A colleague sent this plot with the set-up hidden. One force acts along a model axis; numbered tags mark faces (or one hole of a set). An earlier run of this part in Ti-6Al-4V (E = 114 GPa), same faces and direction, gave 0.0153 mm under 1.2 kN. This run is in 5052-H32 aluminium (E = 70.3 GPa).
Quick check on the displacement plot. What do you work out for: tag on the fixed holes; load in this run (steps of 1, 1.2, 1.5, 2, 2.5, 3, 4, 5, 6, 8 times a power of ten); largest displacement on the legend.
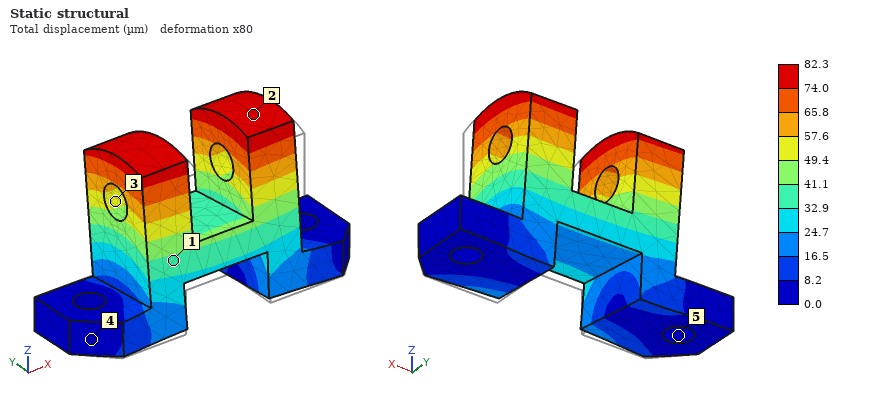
5
4 kN
82.3 µm
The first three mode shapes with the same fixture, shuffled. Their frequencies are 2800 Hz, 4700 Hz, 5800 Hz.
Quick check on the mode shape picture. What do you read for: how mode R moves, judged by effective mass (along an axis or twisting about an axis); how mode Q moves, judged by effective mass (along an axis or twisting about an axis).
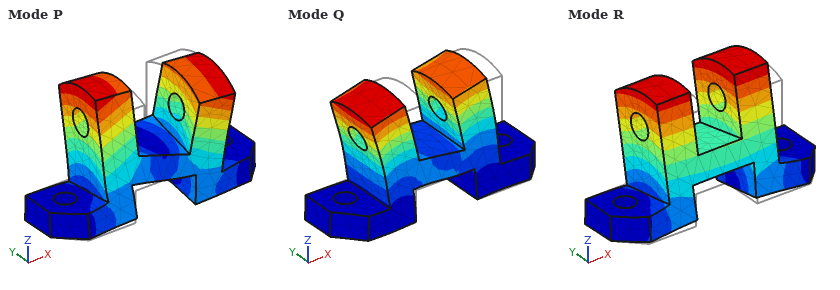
along Y
along X
